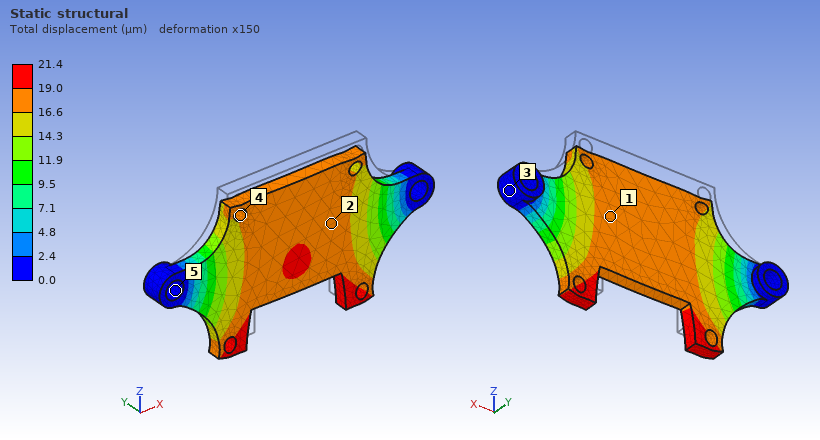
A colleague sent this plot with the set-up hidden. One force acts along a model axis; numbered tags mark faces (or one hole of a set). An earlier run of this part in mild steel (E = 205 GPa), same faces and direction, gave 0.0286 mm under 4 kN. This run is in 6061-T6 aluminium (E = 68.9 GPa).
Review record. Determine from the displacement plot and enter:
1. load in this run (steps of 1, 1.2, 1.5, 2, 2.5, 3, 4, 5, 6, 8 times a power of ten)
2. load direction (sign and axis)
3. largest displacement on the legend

1 kN
-Z
21.4 µm
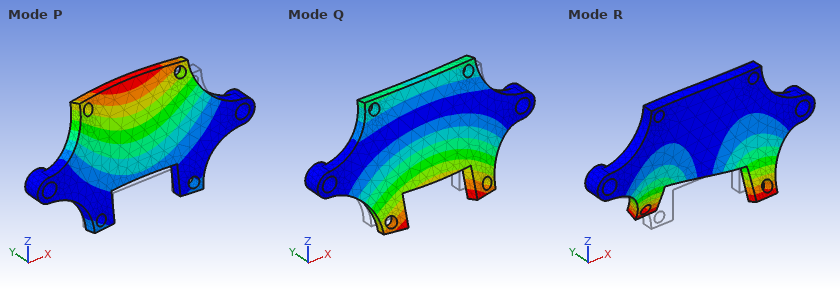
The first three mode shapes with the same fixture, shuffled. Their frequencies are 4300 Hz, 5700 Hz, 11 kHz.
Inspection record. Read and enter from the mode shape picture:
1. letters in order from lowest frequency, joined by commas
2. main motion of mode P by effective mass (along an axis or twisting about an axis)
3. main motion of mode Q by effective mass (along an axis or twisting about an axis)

P, Q, R
along Y
along Y
